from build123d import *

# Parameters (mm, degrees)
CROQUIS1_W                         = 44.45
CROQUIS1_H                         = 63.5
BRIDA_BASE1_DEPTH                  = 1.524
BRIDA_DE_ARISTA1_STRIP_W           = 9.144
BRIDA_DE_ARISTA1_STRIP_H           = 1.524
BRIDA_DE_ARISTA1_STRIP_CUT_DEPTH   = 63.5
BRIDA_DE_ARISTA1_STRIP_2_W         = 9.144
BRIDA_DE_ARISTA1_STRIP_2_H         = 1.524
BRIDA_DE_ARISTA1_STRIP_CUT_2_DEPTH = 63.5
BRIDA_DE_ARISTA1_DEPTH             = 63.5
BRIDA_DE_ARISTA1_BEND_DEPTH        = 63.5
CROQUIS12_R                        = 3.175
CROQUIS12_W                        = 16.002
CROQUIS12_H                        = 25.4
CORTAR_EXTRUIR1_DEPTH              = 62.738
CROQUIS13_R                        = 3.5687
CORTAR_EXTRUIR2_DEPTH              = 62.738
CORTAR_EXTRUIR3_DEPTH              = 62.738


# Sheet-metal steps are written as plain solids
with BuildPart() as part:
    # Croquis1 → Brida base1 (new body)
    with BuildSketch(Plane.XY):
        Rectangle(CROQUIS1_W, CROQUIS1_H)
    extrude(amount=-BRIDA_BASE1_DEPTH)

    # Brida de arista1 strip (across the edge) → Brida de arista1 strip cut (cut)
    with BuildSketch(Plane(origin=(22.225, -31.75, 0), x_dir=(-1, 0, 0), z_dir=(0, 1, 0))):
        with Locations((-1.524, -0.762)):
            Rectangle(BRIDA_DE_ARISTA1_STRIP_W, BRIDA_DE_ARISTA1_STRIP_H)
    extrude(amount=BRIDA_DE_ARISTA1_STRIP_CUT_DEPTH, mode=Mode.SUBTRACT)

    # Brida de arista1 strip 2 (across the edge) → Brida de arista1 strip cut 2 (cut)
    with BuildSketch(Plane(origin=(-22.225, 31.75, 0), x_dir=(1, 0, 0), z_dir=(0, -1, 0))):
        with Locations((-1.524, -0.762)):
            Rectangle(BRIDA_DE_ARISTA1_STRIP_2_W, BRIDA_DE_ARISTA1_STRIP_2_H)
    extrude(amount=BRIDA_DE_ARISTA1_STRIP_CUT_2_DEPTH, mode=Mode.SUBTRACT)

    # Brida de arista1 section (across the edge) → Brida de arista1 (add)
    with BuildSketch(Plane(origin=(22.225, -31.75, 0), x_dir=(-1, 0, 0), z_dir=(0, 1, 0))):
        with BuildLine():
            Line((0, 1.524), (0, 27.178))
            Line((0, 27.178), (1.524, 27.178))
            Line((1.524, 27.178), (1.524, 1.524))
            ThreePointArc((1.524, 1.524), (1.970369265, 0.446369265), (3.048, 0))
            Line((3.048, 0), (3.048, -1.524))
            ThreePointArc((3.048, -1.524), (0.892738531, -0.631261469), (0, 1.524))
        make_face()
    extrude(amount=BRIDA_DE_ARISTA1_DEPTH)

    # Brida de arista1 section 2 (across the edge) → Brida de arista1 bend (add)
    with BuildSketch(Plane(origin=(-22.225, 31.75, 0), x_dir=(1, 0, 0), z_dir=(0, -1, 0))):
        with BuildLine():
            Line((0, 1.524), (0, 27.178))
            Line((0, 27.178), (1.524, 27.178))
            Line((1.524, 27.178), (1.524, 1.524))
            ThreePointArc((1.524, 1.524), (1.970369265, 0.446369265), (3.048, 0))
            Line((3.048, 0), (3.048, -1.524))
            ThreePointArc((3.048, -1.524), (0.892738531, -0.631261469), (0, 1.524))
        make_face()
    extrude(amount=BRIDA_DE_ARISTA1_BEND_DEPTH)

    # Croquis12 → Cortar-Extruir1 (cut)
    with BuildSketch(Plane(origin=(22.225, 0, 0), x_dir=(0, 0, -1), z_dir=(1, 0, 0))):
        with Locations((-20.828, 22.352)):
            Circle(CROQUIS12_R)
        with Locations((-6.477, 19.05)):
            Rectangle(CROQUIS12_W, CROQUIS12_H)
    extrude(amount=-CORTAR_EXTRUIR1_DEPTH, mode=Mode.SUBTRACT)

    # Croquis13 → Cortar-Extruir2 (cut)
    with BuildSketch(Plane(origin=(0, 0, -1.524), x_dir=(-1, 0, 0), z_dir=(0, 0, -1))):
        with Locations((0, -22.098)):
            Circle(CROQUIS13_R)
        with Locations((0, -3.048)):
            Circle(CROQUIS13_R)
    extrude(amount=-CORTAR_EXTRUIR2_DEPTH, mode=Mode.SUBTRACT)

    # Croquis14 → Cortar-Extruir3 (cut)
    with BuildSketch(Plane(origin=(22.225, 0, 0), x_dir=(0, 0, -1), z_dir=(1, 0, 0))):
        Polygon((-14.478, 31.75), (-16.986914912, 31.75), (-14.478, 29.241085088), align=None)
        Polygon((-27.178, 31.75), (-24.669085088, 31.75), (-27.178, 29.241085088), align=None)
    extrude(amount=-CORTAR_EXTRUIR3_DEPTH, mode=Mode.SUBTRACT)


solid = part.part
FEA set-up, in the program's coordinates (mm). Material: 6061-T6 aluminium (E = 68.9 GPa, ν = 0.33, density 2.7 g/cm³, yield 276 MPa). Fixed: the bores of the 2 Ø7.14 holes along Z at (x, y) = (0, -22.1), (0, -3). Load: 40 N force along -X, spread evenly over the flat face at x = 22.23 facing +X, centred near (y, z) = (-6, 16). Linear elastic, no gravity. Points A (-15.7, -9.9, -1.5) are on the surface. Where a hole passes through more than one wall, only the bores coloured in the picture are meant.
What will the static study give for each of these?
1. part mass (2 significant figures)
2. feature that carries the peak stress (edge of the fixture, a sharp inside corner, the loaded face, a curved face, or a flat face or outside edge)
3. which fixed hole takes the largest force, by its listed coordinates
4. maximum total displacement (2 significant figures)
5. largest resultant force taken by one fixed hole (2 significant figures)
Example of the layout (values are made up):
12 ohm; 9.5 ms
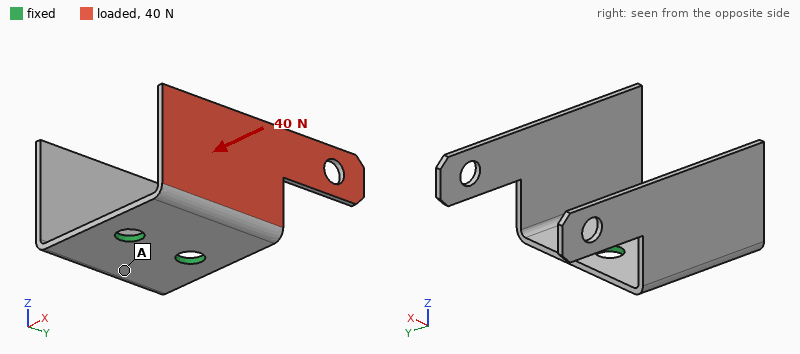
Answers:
17 g; a flat face or outside edge; (0, -3); 0.90 mm; 32 N
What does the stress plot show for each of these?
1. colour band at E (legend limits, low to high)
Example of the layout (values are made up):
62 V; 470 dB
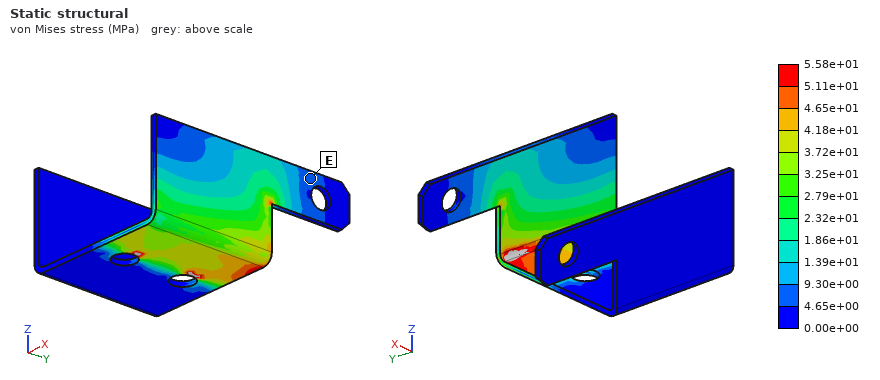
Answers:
4.65e+00 to 9.30e+00 MPa
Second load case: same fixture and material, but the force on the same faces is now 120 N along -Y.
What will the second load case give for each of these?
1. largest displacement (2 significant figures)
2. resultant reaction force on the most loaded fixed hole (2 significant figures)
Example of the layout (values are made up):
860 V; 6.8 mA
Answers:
0.72 mm; 140 N
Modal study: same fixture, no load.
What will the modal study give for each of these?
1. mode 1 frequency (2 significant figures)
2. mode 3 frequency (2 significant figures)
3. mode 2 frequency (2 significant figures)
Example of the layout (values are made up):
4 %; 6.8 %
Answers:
590 Hz; 1000 Hz; 590 Hz
